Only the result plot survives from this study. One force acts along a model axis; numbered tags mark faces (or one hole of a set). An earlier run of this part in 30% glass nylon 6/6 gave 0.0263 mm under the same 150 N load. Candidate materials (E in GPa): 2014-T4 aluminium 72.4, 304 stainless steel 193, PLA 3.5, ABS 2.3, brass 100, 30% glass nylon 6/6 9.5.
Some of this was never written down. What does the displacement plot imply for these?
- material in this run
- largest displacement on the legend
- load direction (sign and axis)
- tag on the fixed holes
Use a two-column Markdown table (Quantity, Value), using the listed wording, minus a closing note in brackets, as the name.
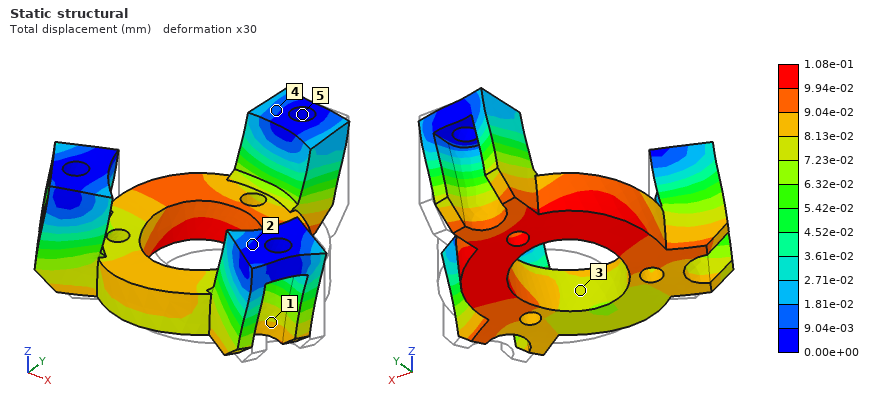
| Quantity | Value |
|---|---|
| material in this run | ABS |
| largest displacement on the legend | 1.08e-01 mm |
| load direction | -X |
| tag on the fixed holes | 5 |
